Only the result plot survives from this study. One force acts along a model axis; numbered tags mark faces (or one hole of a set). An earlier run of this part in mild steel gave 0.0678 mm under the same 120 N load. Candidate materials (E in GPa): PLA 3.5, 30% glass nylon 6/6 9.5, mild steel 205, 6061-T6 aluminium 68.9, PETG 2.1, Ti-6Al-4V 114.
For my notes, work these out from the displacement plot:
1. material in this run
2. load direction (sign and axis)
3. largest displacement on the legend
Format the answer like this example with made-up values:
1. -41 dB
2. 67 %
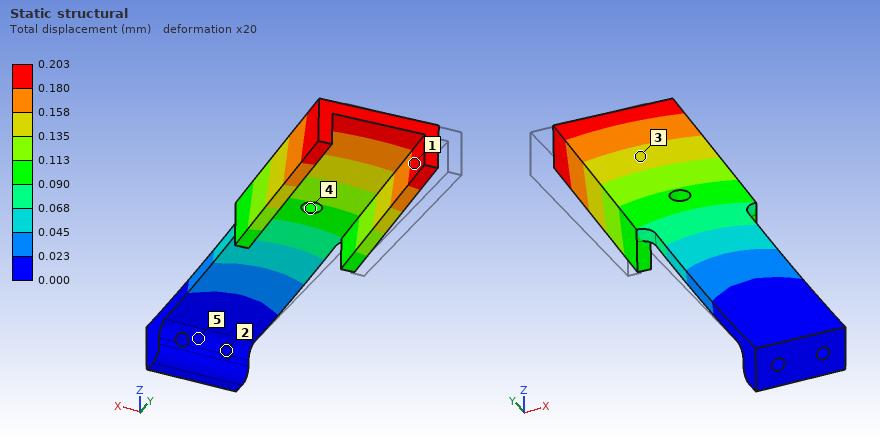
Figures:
1. 6061-T6 aluminium
2. +X
3. 0.203 mm
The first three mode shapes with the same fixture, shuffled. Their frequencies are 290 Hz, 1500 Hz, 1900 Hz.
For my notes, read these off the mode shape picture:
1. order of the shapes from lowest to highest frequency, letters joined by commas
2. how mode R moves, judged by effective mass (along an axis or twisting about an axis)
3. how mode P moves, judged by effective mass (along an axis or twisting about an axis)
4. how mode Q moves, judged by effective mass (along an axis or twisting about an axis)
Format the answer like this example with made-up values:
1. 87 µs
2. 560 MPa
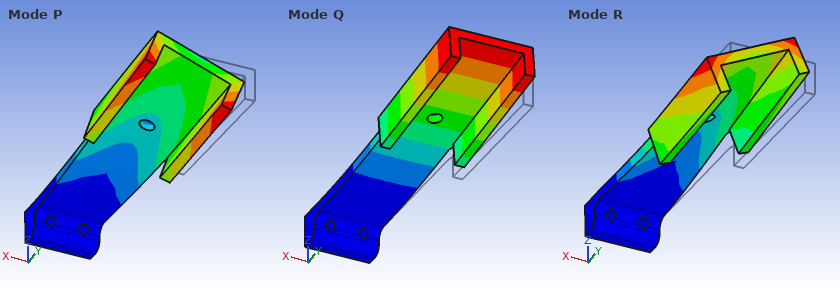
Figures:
1. Q, P, R
2. along X
3. along X
4. along Z
